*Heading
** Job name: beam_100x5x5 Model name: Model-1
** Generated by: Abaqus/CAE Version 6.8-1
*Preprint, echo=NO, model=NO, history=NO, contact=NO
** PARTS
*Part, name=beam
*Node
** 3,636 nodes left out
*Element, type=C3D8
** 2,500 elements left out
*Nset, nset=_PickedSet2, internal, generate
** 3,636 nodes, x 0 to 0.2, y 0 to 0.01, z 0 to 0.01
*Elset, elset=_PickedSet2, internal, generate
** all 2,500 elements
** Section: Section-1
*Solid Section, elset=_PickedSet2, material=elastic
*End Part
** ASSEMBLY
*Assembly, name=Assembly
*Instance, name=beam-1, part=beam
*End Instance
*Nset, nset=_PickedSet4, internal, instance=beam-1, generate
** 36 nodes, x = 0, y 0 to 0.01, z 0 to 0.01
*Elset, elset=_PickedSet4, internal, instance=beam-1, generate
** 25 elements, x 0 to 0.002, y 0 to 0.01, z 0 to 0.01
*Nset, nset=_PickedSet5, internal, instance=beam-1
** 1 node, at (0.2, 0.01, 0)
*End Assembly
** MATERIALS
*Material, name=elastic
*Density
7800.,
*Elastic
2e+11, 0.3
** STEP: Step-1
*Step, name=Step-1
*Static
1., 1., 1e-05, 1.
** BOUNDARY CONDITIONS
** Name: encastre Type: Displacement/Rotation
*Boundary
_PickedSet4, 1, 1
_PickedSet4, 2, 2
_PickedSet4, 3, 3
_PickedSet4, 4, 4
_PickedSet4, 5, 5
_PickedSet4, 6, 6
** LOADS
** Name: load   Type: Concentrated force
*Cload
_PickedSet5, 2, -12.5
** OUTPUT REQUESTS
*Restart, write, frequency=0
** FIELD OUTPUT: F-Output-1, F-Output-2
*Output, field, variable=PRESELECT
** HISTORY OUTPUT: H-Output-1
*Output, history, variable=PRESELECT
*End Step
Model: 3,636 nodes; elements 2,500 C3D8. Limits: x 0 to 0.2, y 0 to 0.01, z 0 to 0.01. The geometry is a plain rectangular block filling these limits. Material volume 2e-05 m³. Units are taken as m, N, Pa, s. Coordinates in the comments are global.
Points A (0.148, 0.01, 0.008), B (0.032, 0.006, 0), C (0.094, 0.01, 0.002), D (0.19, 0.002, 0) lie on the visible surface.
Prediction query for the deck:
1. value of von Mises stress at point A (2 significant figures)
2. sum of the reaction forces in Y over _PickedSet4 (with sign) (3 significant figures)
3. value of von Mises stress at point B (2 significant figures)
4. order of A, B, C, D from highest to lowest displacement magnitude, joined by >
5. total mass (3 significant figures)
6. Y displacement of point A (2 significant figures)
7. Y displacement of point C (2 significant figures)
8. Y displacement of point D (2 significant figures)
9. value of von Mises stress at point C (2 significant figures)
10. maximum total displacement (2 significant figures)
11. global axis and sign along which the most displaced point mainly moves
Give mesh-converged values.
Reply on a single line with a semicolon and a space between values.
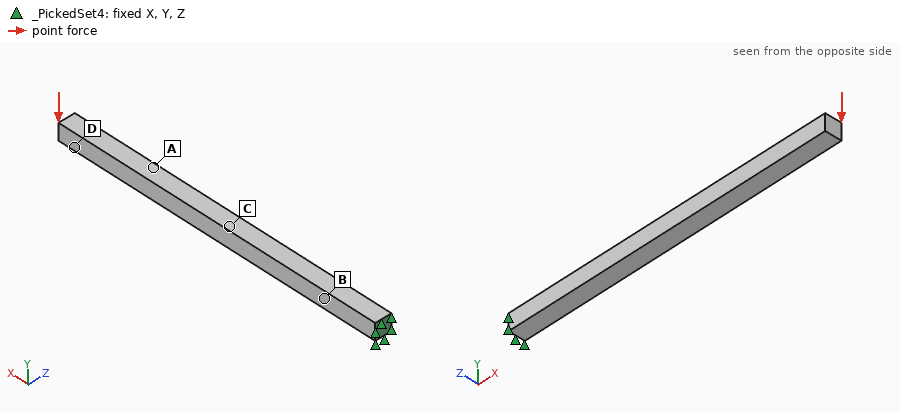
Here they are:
3.9e+06 Pa; 12.5 N; 2.7e+06 Pa; D > A > C > B; 0.156 kg; -1.2e-04 m; -5.6e-05 m; -1.9e-04 m; 8.0e+06 Pa; 2.0e-04 m; -Y
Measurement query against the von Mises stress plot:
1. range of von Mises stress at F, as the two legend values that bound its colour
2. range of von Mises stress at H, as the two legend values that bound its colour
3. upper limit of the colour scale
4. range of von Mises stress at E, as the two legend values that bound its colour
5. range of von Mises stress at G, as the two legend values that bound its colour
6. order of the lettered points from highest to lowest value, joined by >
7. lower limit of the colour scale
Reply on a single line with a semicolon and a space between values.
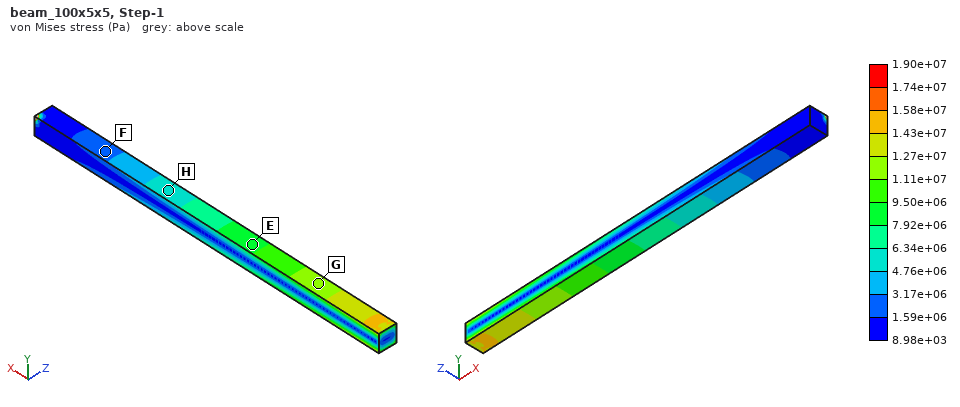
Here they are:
1.59e+06 to 3.17e+06 Pa; 4.76e+06 to 6.34e+06 Pa; 1.90e+07 Pa; 7.92e+06 to 9.50e+06 Pa; 1.11e+07 to 1.27e+07 Pa; G > E > H > F; 8.98e+03 Pa
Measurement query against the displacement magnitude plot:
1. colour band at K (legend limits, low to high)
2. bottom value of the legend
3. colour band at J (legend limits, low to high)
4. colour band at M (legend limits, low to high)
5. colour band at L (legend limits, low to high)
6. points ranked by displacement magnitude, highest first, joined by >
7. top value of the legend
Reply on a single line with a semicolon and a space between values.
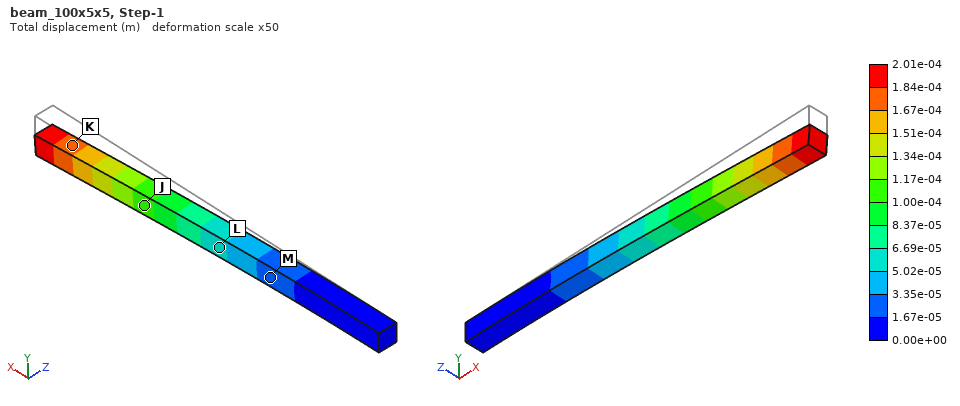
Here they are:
1.67e-04 to 1.84e-04 m; 0.00e+00 m; 1.00e-04 to 1.17e-04 m; 1.67e-05 to 3.35e-05 m; 5.02e-05 to 6.69e-05 m; K > J > L > M; 2.01e-04 m
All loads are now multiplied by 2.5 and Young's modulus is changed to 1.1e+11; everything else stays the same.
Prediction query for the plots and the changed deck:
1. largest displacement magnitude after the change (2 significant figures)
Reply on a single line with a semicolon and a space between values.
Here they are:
9.1e-04 m
